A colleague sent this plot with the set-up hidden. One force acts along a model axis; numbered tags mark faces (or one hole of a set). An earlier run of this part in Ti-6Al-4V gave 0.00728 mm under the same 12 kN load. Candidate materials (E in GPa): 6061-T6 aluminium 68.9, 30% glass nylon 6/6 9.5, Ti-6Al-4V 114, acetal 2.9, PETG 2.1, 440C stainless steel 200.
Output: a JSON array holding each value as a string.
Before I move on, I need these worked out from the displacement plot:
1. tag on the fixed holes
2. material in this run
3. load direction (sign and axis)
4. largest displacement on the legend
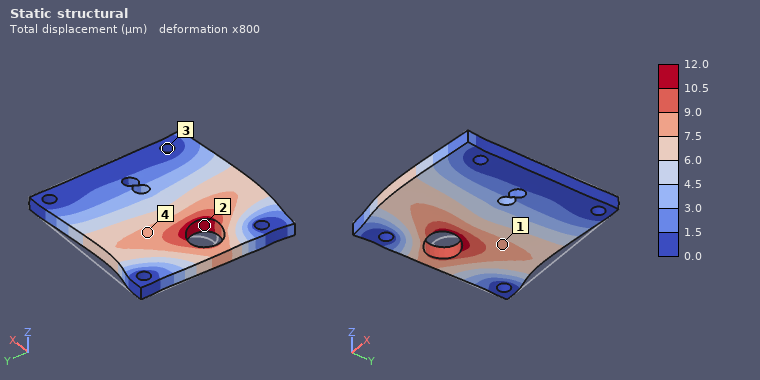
["3", "6061-T6 aluminium", "-Y", "12.0 µm"]
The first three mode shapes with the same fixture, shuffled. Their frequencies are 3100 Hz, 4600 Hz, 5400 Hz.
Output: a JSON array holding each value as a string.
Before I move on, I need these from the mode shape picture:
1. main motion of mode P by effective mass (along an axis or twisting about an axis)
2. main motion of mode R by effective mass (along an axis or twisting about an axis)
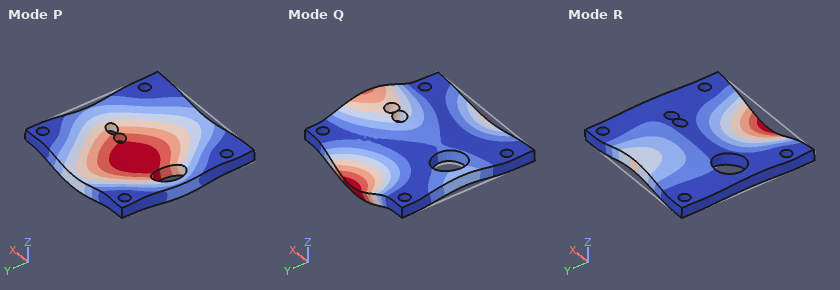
["along Z", "twisting about X"]
